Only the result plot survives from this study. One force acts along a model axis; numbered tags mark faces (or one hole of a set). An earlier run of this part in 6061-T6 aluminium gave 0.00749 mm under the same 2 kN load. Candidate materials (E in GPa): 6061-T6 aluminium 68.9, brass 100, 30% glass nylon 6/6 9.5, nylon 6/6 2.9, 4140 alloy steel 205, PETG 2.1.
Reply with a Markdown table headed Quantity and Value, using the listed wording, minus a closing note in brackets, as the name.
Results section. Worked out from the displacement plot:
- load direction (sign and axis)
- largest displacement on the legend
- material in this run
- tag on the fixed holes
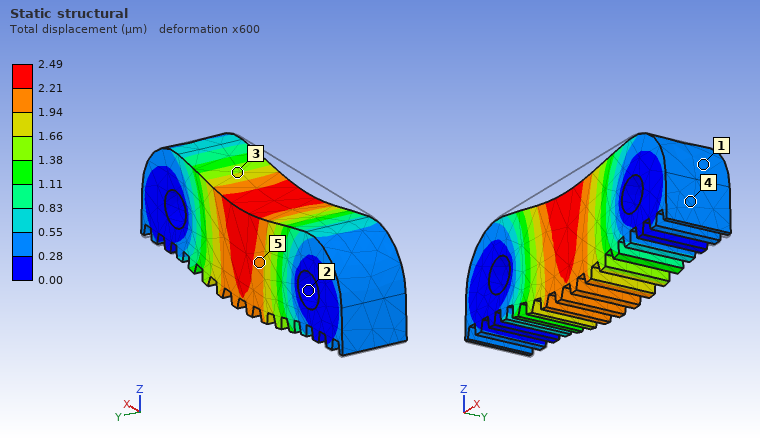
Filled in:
| Quantity | Value |
|---|---|
| load direction | -Z |
| largest displacement on the legend | 2.49 µm |
| material in this run | 4140 alloy steel |
| tag on the fixed holes | 2 |
